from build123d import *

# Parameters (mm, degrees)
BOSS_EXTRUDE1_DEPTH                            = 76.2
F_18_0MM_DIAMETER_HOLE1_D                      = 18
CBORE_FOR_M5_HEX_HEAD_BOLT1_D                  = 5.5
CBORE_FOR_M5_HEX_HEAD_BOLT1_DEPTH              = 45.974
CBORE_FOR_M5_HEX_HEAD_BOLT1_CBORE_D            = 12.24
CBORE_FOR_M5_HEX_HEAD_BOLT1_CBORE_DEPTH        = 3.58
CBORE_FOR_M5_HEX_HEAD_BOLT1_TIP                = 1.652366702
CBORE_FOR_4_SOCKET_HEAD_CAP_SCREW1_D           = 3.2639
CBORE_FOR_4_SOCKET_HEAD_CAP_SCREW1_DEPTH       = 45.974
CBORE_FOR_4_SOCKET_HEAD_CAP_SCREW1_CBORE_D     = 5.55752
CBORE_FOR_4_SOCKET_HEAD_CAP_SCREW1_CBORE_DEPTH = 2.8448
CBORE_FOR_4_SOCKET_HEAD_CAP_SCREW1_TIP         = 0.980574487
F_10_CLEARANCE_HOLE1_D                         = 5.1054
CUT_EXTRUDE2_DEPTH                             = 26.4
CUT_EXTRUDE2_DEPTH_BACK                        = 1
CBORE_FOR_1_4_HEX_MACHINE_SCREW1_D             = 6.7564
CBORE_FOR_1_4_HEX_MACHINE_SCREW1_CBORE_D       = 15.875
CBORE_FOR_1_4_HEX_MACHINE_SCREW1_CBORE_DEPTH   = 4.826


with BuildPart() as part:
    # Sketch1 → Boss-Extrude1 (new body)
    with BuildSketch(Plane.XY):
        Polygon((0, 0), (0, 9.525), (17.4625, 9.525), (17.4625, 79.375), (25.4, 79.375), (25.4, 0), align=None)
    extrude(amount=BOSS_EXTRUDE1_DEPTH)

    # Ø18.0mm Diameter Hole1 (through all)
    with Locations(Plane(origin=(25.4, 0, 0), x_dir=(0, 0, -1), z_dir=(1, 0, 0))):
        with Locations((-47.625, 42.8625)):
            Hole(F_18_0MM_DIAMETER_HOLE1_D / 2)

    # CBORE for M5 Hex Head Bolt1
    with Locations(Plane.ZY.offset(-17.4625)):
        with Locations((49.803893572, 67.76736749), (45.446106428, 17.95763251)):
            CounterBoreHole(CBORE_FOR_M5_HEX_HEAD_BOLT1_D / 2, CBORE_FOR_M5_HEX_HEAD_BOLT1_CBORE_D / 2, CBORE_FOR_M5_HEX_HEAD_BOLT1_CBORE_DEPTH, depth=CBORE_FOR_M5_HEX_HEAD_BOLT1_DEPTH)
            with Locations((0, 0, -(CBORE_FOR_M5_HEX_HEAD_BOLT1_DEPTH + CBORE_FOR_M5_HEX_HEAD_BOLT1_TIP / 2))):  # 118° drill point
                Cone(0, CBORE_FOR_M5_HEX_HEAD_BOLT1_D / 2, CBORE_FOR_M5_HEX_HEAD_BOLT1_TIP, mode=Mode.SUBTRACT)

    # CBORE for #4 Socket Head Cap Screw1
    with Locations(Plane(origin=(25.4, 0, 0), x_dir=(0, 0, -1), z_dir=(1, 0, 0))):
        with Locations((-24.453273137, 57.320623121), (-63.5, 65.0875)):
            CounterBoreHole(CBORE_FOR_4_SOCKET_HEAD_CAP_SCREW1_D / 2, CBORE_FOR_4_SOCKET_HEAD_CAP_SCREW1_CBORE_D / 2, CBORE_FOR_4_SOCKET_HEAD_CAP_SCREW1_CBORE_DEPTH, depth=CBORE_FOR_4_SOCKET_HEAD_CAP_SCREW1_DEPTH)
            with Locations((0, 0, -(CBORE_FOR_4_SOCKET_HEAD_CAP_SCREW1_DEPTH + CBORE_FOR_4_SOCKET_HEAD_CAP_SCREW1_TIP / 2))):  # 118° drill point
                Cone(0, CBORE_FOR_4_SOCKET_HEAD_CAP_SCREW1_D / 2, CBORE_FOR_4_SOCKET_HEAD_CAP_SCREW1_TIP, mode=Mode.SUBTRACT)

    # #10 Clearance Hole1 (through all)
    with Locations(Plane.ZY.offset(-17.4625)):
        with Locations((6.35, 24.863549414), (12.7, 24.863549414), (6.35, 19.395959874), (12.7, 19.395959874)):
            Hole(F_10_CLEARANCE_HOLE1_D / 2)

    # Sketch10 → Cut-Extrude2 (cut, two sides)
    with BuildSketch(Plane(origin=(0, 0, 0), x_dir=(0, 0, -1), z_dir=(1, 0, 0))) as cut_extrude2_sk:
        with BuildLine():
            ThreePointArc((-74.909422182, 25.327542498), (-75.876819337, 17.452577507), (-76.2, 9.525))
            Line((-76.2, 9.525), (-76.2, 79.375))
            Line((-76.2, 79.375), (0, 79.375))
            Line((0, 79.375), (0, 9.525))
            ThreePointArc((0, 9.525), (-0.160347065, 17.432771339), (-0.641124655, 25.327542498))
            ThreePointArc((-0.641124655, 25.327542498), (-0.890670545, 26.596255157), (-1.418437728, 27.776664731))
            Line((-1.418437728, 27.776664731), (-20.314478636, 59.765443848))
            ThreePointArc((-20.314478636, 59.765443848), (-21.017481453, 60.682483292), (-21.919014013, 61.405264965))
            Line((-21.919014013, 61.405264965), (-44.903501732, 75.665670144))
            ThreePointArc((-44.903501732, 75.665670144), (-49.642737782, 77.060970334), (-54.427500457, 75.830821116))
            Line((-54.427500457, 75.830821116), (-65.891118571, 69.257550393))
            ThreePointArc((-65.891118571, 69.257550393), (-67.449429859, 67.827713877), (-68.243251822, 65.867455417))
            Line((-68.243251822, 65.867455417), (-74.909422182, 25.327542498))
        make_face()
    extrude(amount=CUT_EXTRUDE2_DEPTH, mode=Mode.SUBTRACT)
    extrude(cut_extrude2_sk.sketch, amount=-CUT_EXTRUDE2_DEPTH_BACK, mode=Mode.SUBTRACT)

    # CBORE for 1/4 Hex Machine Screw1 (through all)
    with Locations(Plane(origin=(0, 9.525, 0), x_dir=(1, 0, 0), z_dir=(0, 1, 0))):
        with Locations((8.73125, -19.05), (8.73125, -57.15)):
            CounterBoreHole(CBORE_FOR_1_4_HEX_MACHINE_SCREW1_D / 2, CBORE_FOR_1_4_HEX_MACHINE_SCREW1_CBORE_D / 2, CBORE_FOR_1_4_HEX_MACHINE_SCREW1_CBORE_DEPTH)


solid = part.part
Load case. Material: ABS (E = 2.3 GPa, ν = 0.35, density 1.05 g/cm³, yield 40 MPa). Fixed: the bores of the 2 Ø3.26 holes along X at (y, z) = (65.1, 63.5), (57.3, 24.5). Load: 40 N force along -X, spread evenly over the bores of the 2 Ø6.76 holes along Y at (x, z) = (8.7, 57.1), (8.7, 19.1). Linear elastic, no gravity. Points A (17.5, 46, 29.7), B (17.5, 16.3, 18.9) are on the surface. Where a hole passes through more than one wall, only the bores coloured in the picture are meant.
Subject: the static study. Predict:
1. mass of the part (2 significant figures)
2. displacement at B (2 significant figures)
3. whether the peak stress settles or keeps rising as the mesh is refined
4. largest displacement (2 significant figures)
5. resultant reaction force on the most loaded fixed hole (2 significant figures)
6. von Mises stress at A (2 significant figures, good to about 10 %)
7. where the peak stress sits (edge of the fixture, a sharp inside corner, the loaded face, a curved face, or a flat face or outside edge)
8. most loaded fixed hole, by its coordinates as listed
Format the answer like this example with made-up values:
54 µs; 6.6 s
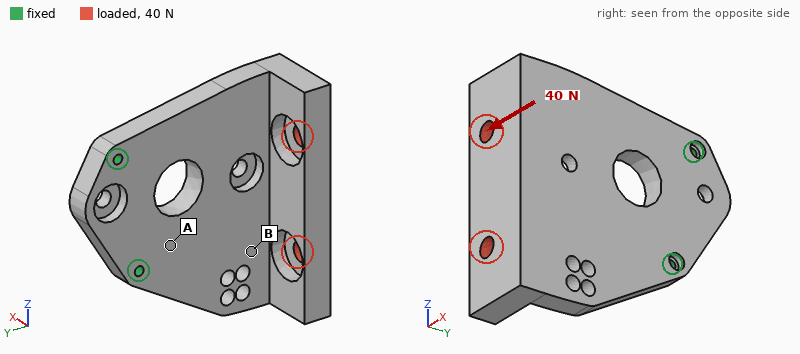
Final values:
45 g; 0.65 mm; keeps rising; 1.2 mm; 36 N; 3.9 MPa; edge of the fixture; (57.3, 24.5)
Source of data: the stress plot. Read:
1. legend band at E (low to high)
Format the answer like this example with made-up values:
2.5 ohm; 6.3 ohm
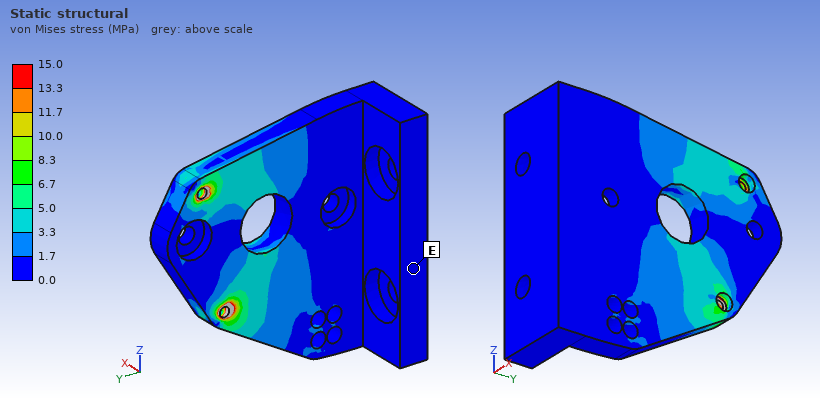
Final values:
0.0 to 1.7 MPa
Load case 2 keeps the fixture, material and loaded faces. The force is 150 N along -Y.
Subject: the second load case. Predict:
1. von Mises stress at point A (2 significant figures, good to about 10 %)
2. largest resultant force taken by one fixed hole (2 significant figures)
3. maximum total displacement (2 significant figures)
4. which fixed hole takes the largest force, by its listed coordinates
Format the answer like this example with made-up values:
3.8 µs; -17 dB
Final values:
4.7 MPa; 97 N; 1.2 mm; (57.3, 24.5)
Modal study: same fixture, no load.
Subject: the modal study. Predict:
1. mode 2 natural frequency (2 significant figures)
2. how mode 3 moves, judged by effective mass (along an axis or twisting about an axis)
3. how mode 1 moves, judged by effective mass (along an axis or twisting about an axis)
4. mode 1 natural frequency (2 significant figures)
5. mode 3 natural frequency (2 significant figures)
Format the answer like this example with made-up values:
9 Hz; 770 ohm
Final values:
530 Hz; along Z; along X; 220 Hz; 1200 Hz
